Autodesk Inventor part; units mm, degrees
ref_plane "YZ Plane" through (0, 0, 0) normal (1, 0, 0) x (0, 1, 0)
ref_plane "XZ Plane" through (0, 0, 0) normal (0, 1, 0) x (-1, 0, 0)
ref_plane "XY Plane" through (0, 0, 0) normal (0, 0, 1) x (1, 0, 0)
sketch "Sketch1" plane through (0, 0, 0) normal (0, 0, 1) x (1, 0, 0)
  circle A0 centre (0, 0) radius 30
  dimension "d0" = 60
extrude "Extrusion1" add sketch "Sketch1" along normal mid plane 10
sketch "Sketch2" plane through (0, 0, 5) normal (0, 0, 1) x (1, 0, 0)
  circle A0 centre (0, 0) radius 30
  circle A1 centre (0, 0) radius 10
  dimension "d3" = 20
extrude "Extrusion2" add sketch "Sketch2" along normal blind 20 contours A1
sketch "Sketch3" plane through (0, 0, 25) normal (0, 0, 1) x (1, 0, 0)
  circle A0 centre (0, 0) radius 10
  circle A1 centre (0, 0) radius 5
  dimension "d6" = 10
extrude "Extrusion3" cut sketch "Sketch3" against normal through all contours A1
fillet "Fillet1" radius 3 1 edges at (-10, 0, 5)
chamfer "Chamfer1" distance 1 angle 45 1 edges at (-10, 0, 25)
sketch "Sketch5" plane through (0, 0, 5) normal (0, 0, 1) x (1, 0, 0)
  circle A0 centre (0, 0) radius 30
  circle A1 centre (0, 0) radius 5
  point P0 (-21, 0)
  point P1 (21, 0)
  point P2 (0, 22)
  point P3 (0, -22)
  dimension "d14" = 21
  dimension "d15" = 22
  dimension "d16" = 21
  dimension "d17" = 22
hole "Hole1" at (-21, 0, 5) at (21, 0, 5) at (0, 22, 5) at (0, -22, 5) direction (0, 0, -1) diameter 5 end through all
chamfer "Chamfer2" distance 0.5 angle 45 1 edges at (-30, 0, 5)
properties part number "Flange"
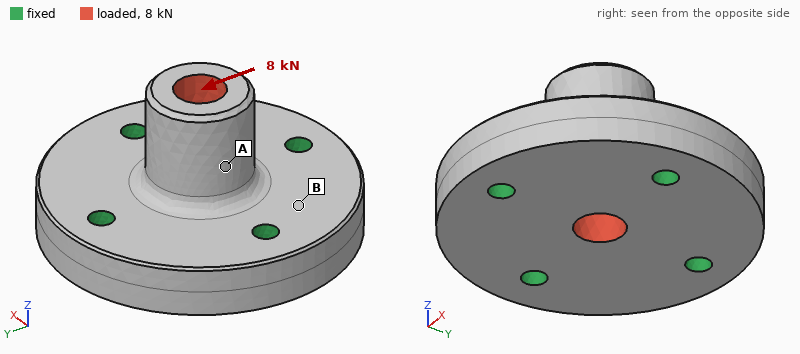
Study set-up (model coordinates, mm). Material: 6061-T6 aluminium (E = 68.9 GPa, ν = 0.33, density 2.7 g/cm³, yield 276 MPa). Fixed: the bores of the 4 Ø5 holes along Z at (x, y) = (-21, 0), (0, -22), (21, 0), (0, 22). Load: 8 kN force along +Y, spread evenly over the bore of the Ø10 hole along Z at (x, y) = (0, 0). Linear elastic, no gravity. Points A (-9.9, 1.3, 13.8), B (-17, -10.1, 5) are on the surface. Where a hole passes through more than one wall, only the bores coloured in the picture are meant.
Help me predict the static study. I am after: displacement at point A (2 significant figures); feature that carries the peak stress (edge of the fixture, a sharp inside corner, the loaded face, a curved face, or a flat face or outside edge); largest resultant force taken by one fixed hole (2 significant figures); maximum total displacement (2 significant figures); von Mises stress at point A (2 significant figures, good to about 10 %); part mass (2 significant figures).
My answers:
20 µm
a curved face
3.2 kN
43 µm
29 MPa
85 g
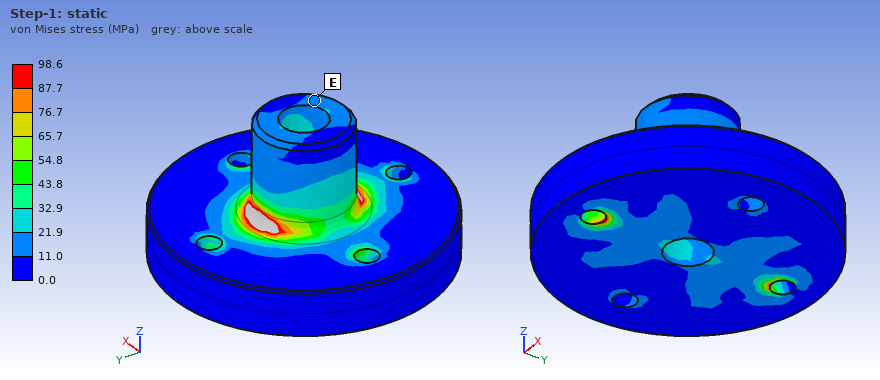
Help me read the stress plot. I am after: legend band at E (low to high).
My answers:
11.0 to 21.9 MPa
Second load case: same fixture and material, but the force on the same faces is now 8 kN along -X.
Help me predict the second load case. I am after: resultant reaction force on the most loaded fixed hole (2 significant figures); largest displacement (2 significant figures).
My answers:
3.4 kN
42 µm
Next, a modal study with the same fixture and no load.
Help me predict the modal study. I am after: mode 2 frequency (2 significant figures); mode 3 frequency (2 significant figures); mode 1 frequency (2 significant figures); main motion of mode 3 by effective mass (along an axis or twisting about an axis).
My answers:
19 kHz
25 kHz
18 kHz
along Z
